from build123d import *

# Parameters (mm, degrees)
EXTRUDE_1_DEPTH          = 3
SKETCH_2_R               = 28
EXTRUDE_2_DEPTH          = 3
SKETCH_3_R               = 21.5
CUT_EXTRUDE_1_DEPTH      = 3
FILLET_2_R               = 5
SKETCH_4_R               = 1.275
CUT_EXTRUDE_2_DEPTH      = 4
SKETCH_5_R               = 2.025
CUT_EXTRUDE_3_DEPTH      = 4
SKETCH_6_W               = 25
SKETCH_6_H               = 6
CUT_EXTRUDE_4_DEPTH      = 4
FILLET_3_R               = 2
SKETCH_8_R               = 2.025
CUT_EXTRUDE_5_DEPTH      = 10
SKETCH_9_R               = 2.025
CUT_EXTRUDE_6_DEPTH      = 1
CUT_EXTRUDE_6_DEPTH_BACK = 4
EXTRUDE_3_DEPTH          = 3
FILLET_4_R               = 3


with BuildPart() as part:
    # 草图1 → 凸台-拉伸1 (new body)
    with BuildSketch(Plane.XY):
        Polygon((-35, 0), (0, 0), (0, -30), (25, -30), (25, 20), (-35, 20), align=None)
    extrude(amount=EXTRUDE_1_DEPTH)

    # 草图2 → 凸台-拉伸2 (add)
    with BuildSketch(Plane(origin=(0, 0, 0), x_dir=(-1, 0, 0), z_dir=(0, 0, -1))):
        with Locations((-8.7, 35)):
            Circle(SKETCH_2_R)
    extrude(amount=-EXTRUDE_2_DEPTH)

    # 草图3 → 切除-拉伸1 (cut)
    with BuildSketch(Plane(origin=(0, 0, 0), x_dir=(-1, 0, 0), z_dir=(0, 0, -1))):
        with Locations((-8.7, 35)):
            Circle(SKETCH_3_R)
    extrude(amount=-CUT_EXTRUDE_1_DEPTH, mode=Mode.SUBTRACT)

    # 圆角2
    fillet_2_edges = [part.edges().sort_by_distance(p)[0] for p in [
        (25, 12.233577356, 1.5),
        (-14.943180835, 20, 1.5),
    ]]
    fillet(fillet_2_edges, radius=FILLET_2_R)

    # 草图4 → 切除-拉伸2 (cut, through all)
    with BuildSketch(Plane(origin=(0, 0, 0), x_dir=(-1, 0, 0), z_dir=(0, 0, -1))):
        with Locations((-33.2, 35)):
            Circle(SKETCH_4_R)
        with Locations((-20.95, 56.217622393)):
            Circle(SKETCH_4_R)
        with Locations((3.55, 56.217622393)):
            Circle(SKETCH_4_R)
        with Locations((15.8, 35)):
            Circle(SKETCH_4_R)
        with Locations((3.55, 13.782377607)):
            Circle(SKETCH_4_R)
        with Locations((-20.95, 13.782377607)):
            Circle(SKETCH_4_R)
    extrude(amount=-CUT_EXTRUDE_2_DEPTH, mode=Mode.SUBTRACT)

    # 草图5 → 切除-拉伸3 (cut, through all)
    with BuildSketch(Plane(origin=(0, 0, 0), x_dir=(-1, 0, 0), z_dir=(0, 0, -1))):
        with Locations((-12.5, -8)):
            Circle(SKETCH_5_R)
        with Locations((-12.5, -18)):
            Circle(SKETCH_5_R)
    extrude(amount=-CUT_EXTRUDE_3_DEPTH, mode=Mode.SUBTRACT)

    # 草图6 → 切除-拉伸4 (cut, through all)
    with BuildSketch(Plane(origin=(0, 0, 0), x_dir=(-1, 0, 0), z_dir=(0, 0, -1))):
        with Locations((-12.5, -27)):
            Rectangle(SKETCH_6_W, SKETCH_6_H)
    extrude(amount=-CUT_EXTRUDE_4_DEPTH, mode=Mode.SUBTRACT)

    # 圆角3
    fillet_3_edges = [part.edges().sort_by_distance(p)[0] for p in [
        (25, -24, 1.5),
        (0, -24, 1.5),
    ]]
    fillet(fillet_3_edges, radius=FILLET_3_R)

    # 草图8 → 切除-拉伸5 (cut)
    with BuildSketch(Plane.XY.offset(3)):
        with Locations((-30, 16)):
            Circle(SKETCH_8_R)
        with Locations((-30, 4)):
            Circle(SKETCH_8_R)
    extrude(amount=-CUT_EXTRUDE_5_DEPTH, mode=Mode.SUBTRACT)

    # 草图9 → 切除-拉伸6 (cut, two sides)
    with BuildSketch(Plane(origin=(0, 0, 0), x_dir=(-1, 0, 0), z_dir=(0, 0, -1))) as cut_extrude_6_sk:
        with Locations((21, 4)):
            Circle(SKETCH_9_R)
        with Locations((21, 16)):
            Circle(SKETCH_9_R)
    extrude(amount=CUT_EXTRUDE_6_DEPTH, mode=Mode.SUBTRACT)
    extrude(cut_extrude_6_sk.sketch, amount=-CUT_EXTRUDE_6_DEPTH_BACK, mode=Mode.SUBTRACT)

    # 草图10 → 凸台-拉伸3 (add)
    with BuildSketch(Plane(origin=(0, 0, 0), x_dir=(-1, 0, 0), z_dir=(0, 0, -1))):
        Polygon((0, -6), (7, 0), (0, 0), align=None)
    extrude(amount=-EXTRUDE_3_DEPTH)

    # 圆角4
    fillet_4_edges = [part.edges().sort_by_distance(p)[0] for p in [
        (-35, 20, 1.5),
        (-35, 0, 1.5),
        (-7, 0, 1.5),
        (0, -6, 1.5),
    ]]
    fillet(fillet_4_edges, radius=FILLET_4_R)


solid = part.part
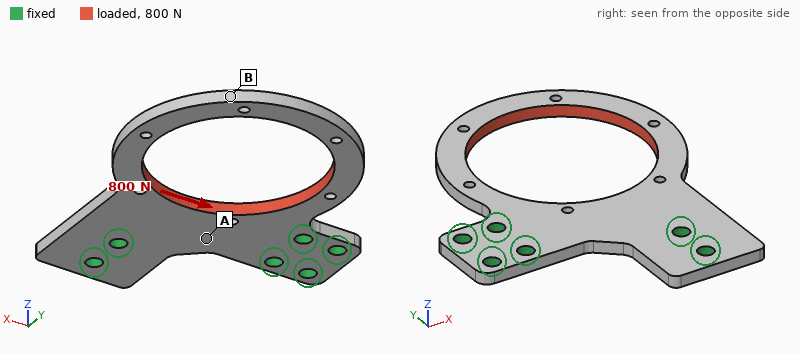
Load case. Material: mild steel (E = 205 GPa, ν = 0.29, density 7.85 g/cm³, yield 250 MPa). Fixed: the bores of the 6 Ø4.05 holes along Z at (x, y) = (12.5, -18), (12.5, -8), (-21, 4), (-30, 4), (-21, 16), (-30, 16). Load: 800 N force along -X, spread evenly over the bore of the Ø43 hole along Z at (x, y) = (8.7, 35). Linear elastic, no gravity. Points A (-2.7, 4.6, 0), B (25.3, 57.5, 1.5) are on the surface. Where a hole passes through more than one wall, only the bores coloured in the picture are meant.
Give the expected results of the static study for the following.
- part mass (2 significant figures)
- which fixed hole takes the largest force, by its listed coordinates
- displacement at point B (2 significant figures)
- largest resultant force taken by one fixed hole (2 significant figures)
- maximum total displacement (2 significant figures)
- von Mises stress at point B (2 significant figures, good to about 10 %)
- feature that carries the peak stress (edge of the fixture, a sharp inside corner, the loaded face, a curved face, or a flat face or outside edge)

55 g
(-21, 16)
97 µm
730 N
98 µm
56 MPa
a curved face
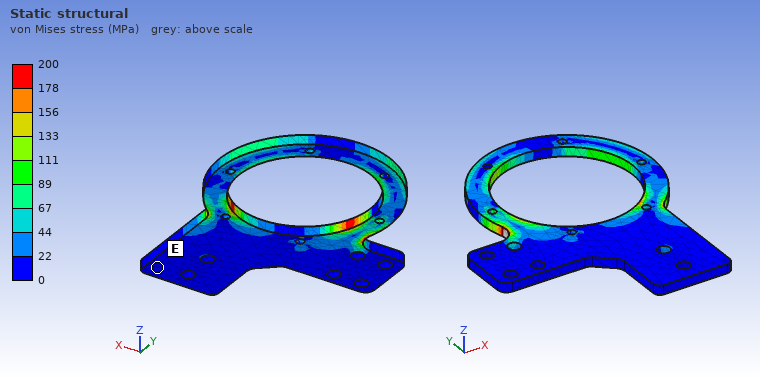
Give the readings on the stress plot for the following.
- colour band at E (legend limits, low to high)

0 to 22 MPa
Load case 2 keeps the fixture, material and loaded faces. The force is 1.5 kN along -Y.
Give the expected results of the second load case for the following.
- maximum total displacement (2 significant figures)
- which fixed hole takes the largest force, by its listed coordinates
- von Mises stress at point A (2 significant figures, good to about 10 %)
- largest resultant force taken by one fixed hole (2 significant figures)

62 µm
(12.5, -8)
11 MPa
790 N
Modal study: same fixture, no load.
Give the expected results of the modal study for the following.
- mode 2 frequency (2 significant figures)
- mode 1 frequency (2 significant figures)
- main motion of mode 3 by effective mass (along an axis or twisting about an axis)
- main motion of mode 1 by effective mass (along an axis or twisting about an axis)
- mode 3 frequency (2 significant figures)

1700 Hz
680 Hz
along X
along Z
3200 Hz
